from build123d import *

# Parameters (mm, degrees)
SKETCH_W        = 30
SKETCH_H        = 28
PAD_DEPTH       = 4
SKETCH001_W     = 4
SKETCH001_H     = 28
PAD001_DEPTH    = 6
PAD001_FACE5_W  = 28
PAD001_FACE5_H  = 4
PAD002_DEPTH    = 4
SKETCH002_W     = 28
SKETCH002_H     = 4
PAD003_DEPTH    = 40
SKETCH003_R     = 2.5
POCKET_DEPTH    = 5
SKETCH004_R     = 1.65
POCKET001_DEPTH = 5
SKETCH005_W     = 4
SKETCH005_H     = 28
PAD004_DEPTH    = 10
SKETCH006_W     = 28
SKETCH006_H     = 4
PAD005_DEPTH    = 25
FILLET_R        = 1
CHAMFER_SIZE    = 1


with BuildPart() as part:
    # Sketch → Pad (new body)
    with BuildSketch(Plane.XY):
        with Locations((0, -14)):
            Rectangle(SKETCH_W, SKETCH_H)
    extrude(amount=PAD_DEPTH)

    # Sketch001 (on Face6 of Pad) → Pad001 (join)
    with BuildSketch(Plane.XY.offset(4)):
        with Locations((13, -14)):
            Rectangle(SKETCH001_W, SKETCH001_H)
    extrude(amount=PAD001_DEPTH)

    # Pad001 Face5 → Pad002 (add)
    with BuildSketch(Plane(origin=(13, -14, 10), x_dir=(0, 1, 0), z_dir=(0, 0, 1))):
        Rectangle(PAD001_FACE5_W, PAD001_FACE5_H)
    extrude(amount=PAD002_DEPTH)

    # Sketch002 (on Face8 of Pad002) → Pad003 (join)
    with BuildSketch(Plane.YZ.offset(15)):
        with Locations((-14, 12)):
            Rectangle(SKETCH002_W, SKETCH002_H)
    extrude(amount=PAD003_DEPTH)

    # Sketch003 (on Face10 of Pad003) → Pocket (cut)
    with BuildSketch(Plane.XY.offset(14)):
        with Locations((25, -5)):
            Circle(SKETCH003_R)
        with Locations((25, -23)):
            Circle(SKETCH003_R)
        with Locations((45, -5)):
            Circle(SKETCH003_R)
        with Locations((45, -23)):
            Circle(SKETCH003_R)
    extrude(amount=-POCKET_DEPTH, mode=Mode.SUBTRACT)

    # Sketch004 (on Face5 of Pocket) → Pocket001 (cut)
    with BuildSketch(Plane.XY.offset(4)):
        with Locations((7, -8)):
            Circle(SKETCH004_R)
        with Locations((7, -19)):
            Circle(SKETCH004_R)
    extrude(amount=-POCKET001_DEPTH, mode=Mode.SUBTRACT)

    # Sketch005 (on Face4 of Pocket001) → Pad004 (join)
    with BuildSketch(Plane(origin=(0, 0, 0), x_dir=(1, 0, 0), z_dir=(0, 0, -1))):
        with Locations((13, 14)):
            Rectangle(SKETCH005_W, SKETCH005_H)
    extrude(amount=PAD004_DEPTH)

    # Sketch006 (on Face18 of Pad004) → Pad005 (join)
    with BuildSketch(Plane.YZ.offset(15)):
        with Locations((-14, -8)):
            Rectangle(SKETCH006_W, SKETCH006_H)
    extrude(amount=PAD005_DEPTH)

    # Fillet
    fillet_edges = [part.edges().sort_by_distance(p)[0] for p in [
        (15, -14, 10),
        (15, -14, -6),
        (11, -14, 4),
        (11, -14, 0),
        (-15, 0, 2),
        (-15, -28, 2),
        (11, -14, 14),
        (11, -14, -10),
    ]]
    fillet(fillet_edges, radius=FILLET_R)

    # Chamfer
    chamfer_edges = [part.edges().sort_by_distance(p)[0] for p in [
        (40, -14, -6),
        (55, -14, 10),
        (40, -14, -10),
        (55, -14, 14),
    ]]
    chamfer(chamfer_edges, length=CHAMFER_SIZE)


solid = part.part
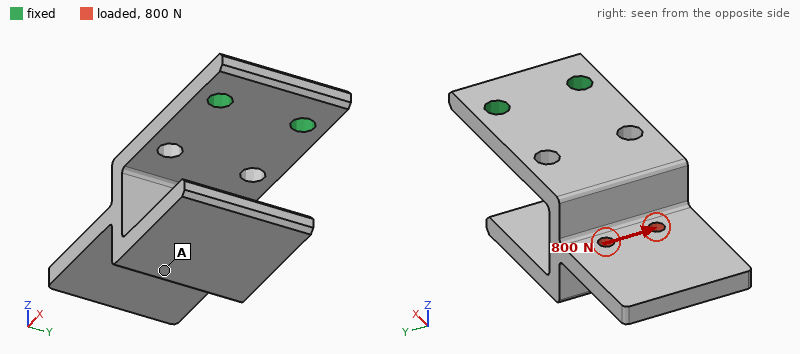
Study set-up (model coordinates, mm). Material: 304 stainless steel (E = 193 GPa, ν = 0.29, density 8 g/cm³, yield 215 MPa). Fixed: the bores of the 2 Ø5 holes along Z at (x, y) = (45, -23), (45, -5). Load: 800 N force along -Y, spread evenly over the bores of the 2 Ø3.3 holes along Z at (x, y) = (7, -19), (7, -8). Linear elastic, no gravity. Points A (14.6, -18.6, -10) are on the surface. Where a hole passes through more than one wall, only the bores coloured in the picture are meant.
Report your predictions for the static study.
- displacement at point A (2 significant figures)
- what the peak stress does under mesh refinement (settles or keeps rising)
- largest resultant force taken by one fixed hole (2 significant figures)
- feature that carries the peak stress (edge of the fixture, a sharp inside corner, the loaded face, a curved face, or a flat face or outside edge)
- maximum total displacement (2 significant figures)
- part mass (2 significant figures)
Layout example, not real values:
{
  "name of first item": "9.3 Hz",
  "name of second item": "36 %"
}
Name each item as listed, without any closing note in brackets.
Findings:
{
  "displacement at point A": "0.10 mm",
  "what the peak stress does under mesh refinement": "keeps rising",
  "largest resultant force taken by one fixed hole": "1.6 kN",
  "feature that carries the peak stress": "edge of the fixture",
  "maximum total displacement": "0.12 mm",
  "part mass": "100 g"
}
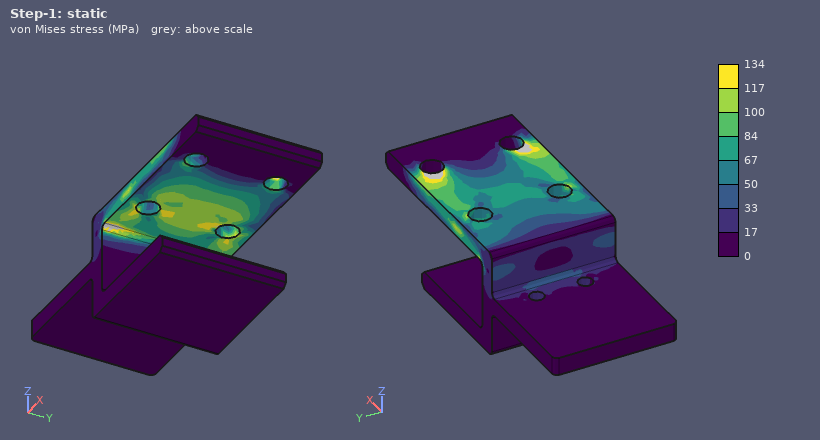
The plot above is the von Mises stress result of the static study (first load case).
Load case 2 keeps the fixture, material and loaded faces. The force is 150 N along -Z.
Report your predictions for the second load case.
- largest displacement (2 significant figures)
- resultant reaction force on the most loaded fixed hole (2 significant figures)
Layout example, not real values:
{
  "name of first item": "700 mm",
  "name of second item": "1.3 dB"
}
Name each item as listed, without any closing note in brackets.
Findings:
{
  "largest displacement": "0.19 mm",
  "resultant reaction force on the most loaded fixed hole": "79 N"
}
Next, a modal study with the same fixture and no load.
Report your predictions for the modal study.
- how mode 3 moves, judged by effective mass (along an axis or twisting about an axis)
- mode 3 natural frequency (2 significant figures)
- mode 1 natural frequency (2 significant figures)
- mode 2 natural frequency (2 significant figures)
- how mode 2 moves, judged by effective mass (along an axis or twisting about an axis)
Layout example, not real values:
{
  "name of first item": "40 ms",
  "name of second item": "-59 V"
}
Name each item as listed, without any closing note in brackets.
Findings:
{
  "how mode 3 moves, judged by effective mass": "along Z",
  "mode 3 natural frequency": "1800 Hz",
  "mode 1 natural frequency": "670 Hz",
  "mode 2 natural frequency": "1500 Hz",
  "how mode 2 moves, judged by effective mass": "along Y"
}
